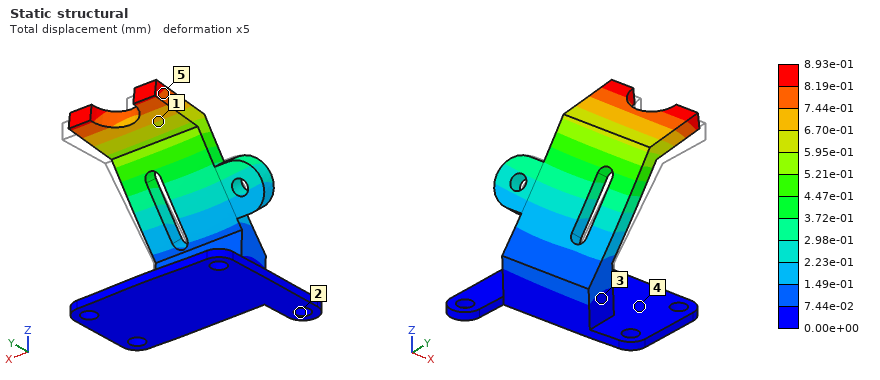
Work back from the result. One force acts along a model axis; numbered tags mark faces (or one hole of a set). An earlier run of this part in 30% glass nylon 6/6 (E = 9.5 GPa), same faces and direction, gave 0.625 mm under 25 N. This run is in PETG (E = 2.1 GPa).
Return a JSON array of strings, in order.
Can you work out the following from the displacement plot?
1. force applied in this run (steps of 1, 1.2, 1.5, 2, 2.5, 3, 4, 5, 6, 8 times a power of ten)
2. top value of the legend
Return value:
["8 N", "8.93e-01 mm"]
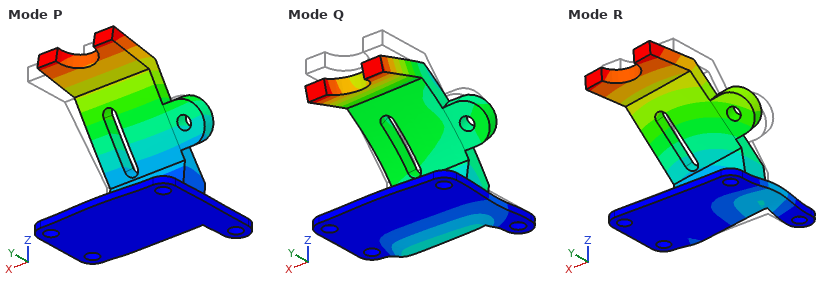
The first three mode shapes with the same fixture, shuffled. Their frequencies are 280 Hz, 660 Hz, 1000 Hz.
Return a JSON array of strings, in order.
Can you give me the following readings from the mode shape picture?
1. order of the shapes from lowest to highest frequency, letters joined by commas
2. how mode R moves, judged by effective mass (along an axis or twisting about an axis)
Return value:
["P, R, Q", "along X"]
